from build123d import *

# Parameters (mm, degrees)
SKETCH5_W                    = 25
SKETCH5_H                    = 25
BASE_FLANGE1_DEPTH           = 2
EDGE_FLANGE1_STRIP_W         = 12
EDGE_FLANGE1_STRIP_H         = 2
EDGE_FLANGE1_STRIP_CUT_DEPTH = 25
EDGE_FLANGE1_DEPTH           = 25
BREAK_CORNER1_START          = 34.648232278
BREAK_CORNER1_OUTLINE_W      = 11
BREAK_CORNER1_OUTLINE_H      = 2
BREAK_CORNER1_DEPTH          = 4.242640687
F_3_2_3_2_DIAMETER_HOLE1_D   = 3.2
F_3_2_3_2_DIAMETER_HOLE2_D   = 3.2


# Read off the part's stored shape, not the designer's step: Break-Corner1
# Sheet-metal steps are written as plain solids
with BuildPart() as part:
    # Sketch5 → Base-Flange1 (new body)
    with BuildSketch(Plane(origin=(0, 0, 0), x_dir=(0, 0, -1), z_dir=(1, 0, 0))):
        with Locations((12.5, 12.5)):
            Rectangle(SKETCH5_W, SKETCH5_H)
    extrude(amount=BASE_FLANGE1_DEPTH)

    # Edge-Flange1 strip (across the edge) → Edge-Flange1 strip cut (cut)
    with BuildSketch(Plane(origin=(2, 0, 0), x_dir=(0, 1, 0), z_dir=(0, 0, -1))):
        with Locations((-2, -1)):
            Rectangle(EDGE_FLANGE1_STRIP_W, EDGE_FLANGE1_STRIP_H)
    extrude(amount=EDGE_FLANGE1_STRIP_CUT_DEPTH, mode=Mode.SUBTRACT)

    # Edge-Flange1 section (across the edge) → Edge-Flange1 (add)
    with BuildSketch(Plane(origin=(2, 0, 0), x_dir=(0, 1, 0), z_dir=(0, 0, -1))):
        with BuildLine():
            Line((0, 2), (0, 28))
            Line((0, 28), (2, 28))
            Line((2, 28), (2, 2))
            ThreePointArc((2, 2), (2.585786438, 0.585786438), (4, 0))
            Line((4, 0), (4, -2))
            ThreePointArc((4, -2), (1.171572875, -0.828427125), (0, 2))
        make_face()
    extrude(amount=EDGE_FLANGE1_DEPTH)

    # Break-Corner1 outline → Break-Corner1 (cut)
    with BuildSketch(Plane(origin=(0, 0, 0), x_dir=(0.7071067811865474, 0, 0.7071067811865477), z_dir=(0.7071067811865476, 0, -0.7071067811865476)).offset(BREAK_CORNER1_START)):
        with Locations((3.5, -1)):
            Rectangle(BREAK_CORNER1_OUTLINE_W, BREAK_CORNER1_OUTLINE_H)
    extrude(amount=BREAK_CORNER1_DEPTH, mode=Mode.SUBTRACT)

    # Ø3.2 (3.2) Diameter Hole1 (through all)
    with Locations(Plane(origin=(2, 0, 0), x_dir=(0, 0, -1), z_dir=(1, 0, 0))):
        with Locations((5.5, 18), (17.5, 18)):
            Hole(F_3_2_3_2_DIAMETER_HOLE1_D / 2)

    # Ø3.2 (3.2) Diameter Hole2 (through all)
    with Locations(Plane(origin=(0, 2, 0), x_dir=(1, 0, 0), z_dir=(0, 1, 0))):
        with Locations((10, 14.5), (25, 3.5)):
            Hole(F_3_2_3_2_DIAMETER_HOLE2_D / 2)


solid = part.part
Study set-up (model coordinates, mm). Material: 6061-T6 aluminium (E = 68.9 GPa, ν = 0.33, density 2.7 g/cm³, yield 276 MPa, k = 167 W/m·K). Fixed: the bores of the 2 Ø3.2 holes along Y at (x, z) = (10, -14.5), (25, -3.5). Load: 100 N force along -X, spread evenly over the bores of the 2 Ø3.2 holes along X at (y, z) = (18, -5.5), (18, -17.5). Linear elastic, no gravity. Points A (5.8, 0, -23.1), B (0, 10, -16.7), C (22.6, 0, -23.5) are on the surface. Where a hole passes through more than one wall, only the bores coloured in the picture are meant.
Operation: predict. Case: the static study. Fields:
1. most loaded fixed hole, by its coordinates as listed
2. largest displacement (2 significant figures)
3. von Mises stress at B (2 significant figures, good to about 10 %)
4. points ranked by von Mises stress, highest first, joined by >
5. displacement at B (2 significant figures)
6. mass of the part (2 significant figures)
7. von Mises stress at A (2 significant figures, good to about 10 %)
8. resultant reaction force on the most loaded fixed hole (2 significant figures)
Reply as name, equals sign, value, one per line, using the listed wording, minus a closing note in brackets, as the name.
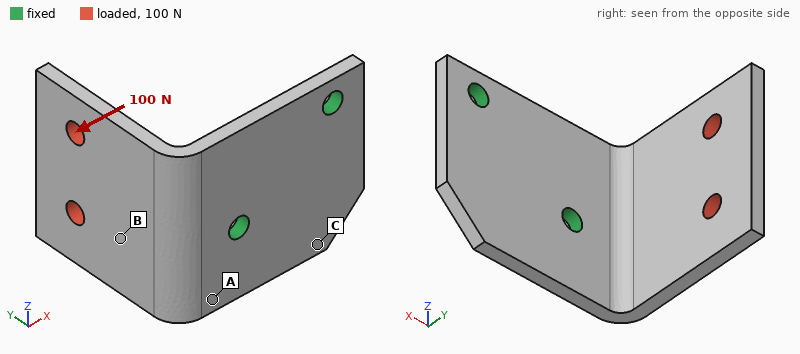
most loaded fixed hole, by its coordinates as listed = (10, -14.5)
largest displacement = 0.51 mm
von Mises stress at B = 44 MPa
points ranked by von Mises stress, highest first, joined by > = A > B > C
displacement at B = 0.17 mm
mass of the part = 6.7 g
von Mises stress at A = 81 MPa
resultant reaction force on the most loaded fixed hole = 81 N
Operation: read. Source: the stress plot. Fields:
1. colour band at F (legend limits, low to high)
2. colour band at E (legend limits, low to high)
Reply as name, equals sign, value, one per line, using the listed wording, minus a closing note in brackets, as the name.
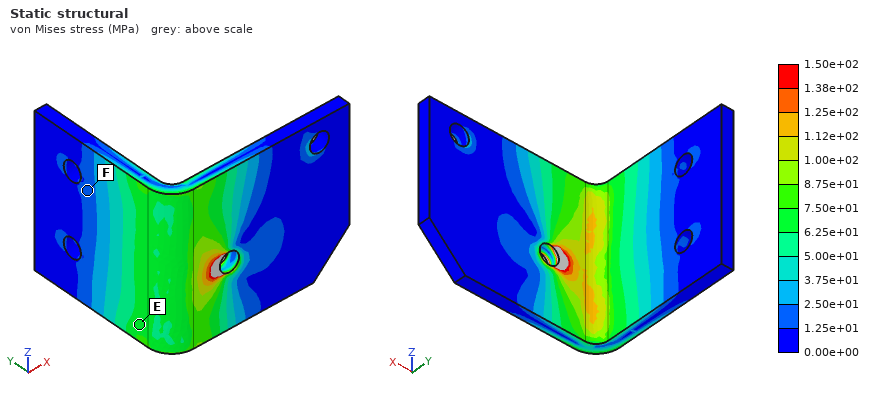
colour band at F = 1.25e+01 to 2.50e+01 MPa
colour band at E = 6.25e+01 to 7.50e+01 MPa
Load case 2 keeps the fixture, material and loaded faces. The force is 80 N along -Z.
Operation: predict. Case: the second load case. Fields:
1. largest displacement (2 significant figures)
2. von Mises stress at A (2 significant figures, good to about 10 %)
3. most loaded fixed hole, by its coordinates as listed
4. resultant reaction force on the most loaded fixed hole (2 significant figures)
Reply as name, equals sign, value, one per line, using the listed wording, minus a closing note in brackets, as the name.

largest displacement = 0.17 mm
von Mises stress at A = 24 MPa
most loaded fixed hole, by its coordinates as listed = (10, -14.5)
resultant reaction force on the most loaded fixed hole = 100 N
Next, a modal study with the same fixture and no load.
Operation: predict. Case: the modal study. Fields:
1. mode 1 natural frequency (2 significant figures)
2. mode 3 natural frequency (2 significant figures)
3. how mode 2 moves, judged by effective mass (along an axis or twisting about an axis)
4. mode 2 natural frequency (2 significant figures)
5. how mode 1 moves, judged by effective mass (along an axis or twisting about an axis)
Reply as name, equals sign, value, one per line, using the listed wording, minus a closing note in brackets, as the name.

mode 1 natural frequency = 1900 Hz
mode 3 natural frequency = 6000 Hz
how mode 2 moves, judged by effective mass = along Z
mode 2 natural frequency = 2700 Hz
how mode 1 moves, judged by effective mass = along X
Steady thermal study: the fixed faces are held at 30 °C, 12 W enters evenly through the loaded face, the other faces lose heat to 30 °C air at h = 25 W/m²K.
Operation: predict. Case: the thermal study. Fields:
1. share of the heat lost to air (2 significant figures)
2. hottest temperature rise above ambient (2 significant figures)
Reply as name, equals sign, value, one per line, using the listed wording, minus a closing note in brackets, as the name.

share of the heat lost to air = 9.2 %
hottest temperature rise above ambient = 41 K
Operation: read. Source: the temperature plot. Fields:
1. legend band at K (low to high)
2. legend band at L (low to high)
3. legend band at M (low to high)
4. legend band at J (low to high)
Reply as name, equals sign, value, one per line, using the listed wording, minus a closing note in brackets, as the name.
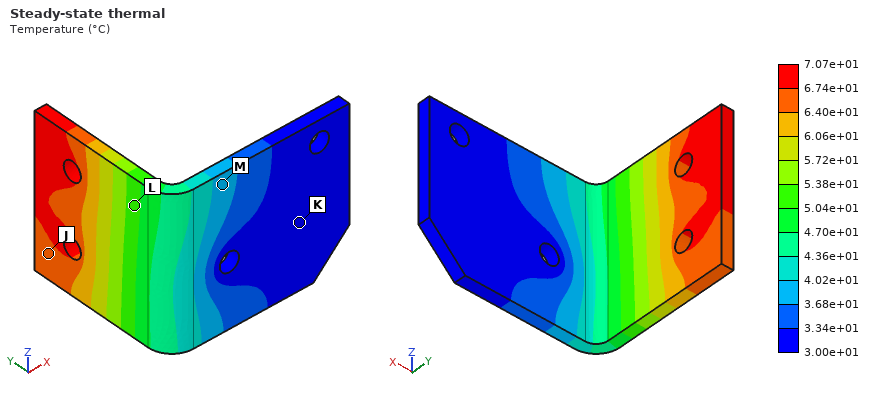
legend band at K = 3.00e+01 to 3.34e+01 °C
legend band at L = 5.04e+01 to 5.38e+01 °C
legend band at M = 3.68e+01 to 4.02e+01 °C
legend band at J = 6.40e+01 to 6.74e+01 °C
